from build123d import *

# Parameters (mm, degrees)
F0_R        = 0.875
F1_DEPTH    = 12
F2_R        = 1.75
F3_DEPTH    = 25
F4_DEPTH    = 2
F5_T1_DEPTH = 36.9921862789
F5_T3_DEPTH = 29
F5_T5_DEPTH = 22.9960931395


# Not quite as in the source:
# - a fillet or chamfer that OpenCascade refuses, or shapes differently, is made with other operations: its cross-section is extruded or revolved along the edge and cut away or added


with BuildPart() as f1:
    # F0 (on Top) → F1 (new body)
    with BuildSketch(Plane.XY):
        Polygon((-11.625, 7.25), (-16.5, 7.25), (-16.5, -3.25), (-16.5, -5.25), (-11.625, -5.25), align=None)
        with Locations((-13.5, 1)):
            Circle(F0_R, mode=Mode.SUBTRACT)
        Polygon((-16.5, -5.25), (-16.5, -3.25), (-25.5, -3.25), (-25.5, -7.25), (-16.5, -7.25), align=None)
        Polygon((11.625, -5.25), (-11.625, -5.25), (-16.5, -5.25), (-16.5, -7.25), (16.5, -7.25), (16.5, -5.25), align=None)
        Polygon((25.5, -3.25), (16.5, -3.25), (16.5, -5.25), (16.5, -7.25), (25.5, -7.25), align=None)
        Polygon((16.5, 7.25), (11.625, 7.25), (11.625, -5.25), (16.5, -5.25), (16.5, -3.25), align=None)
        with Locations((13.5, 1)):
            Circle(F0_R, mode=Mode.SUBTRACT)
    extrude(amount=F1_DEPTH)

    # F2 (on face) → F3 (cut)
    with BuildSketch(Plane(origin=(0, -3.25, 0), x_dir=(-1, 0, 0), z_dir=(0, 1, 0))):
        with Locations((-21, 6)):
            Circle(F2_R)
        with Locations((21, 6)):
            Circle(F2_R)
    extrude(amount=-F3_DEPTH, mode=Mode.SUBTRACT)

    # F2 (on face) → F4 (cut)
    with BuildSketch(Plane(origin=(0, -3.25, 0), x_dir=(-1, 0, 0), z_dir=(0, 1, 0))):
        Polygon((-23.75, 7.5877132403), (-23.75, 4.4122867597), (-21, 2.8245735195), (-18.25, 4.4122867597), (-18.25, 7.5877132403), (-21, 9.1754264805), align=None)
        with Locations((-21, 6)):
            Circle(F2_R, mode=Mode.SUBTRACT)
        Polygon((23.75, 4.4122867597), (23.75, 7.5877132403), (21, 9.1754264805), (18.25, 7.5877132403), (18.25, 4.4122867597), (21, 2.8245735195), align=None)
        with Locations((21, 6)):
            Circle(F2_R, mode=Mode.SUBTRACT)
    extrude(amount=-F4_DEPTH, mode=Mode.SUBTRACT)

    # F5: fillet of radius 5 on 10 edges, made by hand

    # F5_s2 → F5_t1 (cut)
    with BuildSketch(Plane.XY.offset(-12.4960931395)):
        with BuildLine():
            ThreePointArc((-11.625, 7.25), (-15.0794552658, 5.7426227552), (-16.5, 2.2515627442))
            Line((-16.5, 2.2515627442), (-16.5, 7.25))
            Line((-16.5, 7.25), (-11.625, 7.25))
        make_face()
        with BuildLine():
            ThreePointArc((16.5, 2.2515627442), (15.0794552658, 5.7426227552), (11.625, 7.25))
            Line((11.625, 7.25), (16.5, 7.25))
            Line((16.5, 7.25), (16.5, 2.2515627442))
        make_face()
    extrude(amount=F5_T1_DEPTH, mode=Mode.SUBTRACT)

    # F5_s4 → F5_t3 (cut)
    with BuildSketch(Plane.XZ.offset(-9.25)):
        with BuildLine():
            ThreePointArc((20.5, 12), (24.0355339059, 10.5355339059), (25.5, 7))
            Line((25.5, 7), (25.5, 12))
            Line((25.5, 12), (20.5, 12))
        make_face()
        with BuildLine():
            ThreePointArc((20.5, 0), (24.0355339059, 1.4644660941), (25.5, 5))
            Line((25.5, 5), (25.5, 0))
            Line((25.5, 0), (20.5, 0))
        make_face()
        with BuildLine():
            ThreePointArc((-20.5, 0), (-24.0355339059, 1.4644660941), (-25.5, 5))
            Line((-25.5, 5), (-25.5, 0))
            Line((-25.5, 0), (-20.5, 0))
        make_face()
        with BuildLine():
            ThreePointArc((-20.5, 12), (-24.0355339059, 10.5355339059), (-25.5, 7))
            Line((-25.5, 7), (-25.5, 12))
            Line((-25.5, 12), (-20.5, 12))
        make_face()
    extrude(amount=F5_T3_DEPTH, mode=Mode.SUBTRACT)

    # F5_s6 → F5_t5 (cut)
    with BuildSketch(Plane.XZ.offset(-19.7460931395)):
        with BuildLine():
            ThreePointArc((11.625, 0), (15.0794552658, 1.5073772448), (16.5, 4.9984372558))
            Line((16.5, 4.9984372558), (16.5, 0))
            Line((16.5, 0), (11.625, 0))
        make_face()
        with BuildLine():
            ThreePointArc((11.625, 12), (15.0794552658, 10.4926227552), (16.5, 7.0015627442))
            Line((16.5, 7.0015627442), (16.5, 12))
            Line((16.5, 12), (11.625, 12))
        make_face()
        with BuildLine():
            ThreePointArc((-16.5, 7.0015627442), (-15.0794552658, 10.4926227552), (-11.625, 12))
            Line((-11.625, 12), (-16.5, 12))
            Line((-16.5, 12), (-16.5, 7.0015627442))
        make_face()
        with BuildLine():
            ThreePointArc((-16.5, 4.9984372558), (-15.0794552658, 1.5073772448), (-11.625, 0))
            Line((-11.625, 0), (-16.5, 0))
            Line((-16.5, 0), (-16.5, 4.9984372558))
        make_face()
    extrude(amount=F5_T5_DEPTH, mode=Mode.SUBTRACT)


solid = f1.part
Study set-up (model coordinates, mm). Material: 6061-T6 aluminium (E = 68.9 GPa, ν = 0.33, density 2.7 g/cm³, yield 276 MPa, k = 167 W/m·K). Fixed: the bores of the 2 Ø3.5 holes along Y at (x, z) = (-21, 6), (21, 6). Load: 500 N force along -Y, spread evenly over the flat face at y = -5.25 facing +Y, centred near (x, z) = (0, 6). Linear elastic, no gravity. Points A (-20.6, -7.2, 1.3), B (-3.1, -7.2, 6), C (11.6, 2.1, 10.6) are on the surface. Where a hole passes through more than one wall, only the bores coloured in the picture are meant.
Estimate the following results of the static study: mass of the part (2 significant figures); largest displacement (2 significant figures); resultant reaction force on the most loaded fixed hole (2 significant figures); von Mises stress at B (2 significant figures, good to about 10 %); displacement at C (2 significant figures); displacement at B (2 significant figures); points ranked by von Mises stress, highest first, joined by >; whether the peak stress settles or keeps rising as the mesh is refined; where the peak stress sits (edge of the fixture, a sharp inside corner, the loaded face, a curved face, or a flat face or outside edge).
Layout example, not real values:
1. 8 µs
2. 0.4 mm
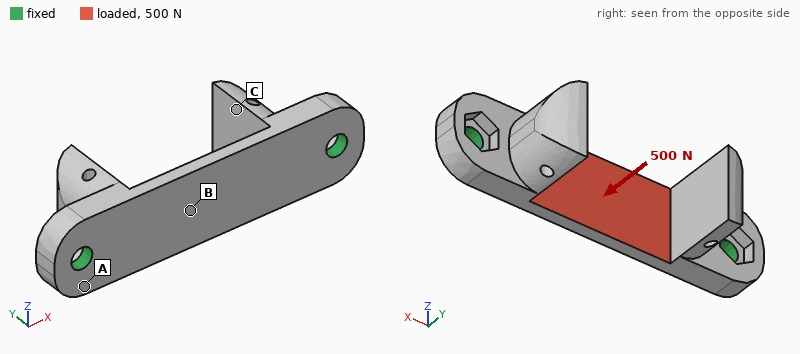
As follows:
1. 6.8 g
2. 0.12 mm
3. 300 N
4. 91 MPa
5. 0.068 mm
6. 0.11 mm
7. B > A > C
8. keeps rising
9. edge of the fixture
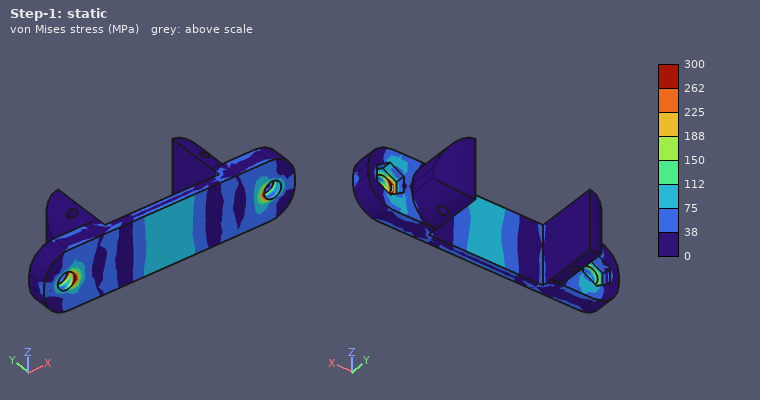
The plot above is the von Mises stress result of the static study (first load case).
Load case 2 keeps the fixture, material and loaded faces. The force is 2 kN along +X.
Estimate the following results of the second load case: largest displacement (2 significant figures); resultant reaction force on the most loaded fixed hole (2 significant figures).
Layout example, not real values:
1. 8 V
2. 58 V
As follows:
1. 15 µm
2. 1.0 kN
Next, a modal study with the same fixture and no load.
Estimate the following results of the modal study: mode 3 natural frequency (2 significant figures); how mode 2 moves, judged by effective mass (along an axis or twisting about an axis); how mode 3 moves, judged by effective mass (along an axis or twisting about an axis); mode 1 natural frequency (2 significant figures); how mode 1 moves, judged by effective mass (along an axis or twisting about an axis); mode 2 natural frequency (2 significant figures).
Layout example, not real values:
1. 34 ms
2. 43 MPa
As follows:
1. 11 kHz
2. along X
3. along Z
4. 6700 Hz
5. along Y
6. 10 kHz
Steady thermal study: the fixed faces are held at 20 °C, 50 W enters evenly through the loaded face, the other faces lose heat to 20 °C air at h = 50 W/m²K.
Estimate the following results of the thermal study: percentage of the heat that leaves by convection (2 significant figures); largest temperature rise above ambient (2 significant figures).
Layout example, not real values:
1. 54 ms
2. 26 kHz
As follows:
1. 5.3 %
2. 71 K
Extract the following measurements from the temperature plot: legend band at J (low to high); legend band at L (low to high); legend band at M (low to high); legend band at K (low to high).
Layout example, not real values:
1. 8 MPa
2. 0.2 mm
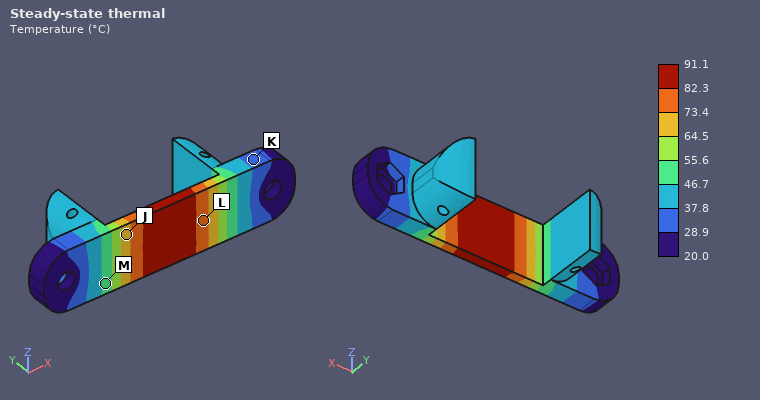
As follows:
1. 64.5 to 73.4 °C
2. 73.4 to 82.3 °C
3. 46.7 to 55.6 °C
4. 28.9 to 37.8 °C
